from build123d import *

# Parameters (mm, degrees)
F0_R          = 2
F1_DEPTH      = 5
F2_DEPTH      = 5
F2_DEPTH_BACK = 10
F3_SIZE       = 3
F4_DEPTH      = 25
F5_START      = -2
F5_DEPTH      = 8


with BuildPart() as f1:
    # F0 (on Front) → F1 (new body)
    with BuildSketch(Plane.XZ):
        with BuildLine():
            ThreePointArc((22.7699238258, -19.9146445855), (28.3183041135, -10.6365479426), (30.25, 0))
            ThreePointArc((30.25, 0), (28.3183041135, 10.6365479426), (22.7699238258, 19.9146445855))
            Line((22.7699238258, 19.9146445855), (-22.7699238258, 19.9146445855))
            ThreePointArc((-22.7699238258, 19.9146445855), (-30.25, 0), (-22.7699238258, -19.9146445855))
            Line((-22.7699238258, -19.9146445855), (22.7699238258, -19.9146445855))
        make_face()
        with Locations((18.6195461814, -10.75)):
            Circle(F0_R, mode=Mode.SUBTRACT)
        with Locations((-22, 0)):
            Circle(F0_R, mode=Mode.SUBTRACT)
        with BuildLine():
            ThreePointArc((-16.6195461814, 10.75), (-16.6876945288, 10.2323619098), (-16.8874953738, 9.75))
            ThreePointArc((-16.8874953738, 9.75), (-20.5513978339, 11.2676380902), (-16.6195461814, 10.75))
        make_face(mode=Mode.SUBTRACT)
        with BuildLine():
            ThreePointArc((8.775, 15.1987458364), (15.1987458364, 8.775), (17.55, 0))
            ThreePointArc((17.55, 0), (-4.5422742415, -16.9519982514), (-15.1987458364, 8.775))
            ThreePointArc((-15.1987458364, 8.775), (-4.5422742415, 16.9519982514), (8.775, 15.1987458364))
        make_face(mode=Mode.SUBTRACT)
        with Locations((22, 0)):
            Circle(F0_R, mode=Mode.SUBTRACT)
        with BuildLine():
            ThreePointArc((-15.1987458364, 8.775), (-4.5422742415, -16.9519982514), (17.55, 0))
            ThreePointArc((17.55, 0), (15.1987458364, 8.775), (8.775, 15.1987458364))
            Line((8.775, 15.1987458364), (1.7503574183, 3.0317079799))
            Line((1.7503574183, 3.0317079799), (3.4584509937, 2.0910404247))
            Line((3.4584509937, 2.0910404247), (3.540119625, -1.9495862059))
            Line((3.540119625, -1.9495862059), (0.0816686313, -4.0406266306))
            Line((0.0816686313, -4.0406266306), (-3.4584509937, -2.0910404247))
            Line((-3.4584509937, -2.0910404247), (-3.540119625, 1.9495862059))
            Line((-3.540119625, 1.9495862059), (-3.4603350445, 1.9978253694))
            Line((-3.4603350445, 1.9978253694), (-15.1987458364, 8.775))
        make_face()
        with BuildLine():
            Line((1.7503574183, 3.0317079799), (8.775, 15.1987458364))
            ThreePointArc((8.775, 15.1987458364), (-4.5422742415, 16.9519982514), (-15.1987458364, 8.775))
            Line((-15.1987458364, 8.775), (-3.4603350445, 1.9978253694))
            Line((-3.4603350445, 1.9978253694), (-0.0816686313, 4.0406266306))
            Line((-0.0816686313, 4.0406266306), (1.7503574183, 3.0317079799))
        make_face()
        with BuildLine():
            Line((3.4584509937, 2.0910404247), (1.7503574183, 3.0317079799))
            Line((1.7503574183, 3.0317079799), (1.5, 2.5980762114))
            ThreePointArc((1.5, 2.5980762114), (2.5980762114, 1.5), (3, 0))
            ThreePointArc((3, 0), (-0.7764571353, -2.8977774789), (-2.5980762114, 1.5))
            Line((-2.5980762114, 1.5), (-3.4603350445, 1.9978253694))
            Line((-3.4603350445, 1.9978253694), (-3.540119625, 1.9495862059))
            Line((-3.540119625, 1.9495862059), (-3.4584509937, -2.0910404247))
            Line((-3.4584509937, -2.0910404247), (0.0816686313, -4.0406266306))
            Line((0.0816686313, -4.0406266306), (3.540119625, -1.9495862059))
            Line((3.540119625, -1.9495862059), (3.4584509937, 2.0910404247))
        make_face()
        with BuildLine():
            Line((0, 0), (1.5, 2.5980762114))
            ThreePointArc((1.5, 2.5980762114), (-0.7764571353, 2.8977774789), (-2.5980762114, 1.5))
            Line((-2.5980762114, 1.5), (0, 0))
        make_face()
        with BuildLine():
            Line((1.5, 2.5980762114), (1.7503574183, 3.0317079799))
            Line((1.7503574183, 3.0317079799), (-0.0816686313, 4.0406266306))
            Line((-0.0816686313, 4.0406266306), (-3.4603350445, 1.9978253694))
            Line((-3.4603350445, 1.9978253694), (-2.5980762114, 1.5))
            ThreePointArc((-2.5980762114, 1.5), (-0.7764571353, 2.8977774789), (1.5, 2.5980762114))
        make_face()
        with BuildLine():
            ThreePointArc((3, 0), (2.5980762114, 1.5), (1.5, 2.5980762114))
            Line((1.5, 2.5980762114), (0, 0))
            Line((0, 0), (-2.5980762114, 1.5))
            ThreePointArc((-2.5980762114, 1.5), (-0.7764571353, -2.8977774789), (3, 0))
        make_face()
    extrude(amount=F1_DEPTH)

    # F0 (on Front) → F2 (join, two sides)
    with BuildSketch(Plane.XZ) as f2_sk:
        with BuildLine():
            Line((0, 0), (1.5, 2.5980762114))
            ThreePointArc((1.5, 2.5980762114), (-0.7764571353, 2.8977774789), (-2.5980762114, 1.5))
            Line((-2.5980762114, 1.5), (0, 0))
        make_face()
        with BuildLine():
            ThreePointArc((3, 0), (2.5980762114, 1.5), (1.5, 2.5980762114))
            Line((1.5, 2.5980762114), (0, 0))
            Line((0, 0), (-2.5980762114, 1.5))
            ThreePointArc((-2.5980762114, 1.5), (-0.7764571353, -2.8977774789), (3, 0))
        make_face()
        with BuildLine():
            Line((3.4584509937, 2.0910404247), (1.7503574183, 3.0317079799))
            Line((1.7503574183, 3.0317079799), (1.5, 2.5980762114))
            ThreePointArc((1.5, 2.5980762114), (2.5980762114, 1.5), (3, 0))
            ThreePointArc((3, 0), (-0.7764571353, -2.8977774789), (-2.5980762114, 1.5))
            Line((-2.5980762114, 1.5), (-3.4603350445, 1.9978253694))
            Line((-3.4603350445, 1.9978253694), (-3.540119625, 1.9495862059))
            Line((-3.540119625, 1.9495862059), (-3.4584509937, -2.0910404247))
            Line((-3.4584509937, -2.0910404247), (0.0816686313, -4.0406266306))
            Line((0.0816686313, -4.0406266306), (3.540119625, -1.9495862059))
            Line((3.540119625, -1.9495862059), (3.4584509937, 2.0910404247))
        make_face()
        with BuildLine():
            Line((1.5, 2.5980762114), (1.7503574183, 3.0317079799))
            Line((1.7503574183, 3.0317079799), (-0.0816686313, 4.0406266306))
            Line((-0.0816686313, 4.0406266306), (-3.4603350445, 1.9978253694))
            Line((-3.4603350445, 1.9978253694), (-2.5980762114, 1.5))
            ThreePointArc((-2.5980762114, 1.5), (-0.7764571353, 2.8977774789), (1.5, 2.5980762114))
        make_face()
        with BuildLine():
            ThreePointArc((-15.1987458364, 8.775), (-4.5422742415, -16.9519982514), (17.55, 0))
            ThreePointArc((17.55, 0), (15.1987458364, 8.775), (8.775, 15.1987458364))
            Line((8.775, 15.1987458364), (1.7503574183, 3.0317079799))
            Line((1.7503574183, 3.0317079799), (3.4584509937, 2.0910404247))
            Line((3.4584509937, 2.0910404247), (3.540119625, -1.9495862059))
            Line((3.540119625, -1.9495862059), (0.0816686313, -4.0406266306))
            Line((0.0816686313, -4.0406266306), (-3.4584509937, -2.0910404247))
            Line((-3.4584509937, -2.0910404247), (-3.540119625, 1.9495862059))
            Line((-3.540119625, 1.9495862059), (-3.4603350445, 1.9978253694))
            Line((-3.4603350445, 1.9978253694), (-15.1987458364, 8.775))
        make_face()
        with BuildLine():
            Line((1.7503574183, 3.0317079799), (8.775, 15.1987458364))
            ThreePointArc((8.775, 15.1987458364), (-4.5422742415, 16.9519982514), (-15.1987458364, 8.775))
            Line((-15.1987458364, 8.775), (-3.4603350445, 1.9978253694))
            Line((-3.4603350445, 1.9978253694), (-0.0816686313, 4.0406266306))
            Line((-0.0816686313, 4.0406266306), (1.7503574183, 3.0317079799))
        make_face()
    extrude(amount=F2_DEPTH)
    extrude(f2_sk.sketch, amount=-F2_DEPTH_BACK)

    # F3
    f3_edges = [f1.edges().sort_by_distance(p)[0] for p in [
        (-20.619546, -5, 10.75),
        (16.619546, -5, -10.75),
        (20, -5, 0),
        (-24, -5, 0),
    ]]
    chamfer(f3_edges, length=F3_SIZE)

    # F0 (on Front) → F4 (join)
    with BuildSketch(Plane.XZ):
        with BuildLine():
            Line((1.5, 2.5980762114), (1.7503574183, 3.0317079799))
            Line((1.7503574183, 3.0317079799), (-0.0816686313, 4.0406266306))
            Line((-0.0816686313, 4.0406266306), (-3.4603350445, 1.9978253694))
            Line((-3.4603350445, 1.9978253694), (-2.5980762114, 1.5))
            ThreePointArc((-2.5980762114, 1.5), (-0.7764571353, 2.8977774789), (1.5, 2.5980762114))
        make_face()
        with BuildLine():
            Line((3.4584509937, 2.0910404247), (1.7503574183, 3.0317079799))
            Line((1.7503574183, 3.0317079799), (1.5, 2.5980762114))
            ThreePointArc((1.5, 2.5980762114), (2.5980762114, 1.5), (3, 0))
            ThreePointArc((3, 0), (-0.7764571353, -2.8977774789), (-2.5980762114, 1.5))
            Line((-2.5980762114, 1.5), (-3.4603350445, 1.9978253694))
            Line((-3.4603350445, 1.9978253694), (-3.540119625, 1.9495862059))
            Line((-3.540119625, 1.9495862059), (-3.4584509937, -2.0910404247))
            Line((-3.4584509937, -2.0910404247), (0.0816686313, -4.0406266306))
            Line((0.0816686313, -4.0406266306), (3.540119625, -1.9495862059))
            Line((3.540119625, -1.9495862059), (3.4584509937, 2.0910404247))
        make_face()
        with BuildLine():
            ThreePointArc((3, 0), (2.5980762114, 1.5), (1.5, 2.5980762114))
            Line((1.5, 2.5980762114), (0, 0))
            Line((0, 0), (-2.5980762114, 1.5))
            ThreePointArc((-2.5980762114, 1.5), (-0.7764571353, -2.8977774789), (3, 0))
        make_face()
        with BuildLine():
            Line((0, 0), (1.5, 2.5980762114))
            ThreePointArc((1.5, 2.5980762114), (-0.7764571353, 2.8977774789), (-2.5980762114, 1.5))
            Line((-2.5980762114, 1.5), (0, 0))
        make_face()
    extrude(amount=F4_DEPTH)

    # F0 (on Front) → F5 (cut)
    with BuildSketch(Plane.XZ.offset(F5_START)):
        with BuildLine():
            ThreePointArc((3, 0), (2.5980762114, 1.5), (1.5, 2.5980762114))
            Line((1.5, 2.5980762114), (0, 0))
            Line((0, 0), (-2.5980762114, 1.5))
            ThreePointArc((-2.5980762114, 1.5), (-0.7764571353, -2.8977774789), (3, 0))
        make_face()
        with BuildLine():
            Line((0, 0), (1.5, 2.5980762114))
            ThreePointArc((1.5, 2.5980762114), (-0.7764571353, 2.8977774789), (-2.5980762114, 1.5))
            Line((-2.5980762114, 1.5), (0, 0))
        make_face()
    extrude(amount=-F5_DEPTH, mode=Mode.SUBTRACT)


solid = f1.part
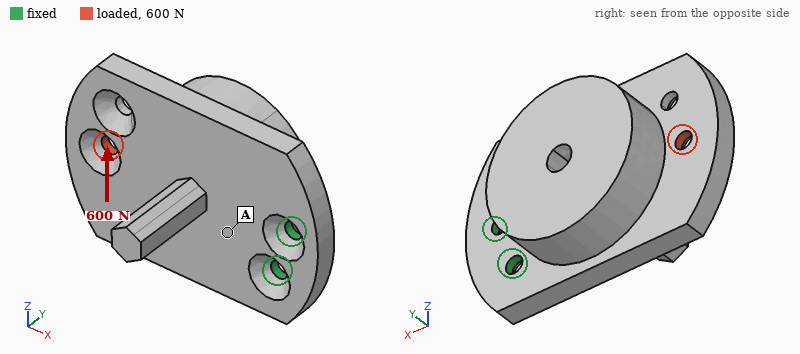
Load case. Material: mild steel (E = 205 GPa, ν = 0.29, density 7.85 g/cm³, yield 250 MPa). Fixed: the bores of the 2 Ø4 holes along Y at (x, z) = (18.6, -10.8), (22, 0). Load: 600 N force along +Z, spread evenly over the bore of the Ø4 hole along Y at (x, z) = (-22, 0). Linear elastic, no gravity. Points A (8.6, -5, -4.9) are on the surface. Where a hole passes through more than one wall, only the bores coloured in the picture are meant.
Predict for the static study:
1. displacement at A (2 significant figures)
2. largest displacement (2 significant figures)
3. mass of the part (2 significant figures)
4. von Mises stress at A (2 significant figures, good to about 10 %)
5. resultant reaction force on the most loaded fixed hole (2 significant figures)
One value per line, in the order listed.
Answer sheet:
3.3 µm
17 µm
160 g
15 MPa
1.9 kN
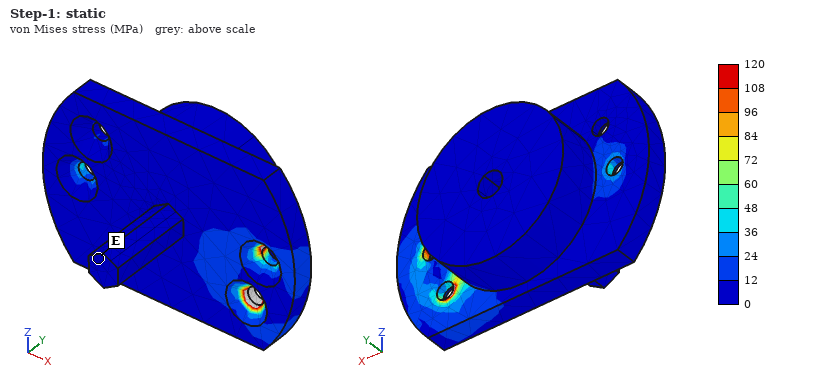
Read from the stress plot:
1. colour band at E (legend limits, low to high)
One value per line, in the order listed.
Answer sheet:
0 to 12 MPa
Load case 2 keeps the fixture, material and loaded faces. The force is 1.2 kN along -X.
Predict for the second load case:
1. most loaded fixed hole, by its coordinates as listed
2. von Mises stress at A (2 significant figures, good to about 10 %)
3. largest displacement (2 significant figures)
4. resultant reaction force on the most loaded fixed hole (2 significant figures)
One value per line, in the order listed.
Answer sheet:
(22, 0)
7.2 MPa
8.7 µm
1.0 kN
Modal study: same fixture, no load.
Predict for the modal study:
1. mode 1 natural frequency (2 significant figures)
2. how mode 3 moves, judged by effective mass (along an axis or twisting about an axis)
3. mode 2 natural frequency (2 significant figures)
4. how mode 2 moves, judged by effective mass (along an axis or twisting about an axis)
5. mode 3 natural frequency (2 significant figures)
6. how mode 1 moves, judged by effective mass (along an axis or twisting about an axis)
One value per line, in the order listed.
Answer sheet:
1100 Hz
twisting about X
4200 Hz
along Z
5000 Hz
along Y
